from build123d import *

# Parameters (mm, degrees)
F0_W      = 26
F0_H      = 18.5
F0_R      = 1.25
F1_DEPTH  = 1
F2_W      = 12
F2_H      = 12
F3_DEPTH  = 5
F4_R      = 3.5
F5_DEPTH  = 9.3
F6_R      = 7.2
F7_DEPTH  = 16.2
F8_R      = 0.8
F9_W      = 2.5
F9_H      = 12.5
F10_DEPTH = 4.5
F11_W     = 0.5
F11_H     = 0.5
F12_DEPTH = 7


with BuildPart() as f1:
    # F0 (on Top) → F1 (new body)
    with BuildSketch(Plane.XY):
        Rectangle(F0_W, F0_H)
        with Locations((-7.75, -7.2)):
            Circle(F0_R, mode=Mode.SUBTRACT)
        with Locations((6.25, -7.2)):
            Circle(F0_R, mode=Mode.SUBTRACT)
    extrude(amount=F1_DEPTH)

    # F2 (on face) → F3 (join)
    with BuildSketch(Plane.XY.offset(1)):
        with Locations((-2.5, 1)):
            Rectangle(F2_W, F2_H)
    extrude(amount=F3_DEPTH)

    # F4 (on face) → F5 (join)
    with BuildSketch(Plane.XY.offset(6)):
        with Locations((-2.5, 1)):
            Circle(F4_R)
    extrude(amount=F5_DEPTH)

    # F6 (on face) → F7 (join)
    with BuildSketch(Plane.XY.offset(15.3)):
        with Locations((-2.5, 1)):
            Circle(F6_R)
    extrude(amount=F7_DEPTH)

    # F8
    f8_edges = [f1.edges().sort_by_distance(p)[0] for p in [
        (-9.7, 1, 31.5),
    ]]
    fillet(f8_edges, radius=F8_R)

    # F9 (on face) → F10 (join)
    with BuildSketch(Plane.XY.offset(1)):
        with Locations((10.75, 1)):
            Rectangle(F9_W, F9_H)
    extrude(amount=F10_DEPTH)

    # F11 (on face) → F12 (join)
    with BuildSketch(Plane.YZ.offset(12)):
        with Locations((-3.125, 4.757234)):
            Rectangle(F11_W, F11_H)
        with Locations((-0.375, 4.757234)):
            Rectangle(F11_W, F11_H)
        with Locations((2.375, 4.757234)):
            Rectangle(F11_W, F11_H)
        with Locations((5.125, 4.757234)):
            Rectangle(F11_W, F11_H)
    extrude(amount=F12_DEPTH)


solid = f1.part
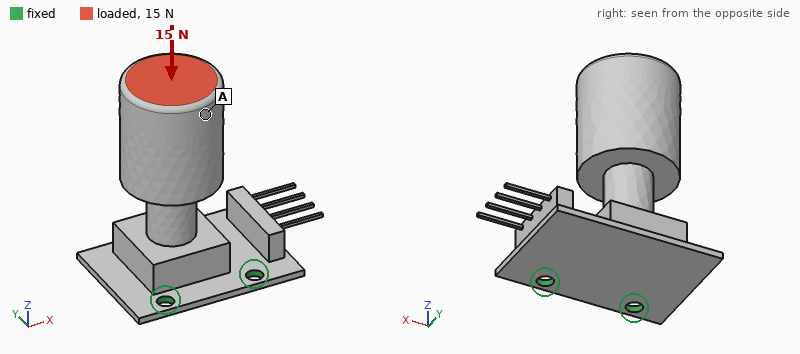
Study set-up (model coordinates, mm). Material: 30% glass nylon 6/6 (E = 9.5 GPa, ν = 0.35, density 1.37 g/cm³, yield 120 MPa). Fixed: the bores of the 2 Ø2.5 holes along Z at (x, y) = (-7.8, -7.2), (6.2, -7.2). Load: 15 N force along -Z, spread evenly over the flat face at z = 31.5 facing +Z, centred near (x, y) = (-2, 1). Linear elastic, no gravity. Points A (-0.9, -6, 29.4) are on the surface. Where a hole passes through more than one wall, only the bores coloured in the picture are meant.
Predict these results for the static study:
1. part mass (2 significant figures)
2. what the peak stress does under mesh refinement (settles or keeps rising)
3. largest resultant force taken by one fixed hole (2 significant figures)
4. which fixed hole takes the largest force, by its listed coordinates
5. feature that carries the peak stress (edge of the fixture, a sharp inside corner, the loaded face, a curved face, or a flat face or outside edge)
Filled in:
5.9 g
keeps rising
8.7 N
(-7.8, -7.2)
edge of the fixture
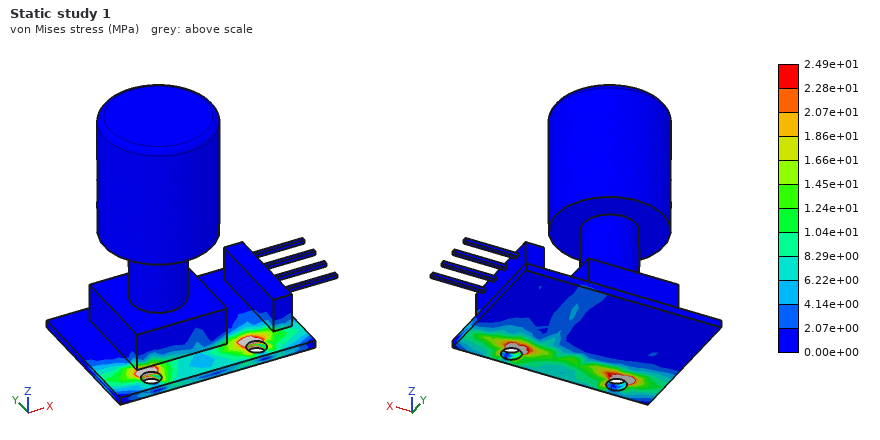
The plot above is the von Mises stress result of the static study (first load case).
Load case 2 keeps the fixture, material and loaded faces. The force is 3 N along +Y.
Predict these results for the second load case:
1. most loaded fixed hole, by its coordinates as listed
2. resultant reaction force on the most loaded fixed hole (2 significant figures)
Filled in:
(-7.8, -7.2)
2.4 N
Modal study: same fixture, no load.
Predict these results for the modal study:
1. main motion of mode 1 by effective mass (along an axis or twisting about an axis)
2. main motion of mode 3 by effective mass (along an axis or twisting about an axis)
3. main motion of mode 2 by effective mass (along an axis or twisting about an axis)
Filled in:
along Y
along Z
along X
